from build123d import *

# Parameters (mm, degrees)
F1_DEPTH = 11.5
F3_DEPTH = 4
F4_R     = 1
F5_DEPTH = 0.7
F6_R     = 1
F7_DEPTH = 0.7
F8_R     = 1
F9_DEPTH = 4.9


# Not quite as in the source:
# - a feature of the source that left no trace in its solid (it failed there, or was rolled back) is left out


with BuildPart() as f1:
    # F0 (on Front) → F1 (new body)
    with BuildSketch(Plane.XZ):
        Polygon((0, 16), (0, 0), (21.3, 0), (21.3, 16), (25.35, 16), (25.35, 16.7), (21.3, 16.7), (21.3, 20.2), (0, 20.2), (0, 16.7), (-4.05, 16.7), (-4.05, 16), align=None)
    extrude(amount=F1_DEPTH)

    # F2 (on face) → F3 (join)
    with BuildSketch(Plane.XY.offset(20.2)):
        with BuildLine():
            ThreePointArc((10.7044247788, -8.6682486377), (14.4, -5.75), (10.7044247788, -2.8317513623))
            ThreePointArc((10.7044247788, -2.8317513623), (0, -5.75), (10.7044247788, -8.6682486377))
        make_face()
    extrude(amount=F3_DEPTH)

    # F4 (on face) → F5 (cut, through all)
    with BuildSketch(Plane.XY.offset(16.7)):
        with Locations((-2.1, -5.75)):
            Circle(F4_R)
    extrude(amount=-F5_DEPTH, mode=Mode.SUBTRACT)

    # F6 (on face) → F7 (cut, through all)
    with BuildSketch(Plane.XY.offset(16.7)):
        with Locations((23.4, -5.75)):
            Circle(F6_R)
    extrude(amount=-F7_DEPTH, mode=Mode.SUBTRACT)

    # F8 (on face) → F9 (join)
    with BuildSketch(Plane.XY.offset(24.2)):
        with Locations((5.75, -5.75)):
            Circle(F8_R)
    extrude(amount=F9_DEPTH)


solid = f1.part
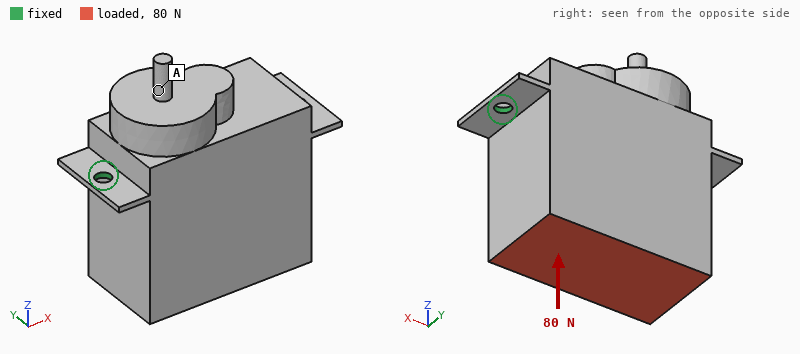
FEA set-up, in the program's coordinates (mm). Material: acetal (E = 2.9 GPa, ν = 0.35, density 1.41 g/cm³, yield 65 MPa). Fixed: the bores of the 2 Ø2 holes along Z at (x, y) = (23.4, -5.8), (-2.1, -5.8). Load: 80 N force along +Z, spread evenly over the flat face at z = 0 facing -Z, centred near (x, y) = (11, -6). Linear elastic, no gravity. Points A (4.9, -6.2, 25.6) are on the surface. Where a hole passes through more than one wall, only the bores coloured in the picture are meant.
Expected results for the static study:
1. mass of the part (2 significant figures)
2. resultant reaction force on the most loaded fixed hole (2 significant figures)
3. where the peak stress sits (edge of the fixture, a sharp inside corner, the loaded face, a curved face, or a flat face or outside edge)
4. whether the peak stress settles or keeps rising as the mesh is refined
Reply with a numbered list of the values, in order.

1. 7.8 g
2. 40 N
3. edge of the fixture
4. keeps rising
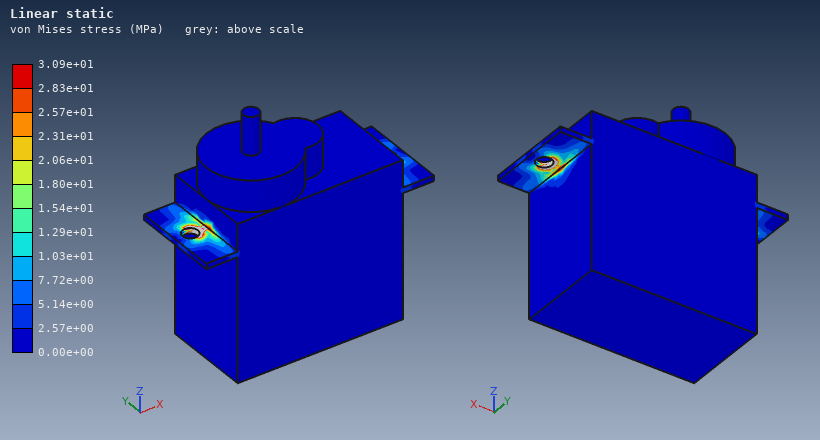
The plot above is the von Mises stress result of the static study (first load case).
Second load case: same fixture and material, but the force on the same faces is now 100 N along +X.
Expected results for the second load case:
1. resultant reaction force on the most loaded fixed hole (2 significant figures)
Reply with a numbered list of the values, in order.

1. 88 N
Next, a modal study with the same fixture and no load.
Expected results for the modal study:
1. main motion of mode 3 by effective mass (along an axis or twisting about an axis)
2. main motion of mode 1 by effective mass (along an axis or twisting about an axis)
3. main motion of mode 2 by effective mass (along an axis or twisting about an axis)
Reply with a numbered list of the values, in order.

1. along X
2. along Y
3. along Z
